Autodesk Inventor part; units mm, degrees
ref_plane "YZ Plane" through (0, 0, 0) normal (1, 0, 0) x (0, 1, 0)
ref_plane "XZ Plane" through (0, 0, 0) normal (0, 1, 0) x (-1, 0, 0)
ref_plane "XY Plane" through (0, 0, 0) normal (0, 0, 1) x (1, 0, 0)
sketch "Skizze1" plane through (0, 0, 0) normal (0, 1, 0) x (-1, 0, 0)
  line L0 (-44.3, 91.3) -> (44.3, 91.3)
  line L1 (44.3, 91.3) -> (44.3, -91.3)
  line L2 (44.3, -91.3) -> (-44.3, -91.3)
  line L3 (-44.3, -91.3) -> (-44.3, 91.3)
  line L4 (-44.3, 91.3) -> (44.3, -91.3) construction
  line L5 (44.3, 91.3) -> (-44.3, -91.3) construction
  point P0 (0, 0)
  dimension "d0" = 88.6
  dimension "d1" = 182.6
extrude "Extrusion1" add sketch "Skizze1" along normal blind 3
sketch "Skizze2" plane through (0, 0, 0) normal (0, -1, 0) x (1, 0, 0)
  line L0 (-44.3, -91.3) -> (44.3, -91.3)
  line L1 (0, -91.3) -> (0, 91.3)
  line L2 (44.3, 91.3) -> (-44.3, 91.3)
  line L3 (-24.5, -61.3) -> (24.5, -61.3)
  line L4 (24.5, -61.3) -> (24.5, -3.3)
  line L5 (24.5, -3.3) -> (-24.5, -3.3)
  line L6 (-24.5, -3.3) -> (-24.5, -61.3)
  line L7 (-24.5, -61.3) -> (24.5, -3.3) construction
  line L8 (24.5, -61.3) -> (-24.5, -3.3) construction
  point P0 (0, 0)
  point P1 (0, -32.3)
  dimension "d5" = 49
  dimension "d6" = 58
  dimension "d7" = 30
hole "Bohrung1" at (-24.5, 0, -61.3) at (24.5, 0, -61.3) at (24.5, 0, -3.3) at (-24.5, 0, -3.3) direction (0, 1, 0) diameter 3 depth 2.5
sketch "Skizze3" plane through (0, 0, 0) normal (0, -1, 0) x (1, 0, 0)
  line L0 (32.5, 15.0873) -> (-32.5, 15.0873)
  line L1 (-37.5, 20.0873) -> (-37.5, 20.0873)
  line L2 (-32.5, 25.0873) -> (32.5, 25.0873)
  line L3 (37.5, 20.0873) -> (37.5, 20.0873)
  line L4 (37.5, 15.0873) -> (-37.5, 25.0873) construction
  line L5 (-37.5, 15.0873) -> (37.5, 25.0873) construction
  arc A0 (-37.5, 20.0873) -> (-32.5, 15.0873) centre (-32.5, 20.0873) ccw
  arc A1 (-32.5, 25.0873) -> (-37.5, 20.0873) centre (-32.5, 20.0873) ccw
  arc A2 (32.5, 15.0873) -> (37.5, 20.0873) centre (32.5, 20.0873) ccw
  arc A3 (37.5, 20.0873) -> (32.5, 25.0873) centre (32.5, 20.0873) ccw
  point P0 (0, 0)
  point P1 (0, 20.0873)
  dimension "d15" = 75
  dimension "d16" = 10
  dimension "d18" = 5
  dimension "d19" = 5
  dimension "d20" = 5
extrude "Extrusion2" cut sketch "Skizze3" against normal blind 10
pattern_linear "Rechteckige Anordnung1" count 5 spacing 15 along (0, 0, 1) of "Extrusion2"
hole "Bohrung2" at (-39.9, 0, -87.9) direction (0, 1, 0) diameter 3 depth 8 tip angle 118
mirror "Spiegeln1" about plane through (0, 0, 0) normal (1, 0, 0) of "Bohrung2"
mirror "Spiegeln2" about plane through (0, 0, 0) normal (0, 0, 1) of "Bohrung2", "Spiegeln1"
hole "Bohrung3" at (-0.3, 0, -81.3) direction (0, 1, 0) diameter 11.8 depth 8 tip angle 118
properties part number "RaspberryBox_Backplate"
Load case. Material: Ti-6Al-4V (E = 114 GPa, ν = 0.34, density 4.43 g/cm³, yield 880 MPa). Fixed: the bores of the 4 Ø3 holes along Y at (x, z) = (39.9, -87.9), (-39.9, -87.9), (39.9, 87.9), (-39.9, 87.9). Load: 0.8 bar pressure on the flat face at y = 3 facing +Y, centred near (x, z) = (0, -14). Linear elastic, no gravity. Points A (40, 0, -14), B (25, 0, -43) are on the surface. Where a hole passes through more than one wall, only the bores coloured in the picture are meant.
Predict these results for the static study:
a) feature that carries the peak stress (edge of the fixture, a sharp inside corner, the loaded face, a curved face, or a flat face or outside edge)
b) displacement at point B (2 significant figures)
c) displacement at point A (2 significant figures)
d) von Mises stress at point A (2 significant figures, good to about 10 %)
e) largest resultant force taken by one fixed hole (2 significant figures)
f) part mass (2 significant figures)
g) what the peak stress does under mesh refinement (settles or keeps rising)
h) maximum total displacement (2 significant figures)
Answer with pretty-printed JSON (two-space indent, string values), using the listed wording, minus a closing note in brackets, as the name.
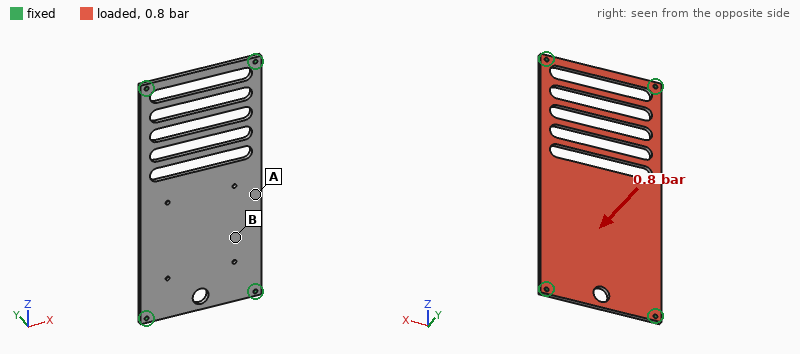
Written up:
{
  "feature that carries the peak stress": "edge of the fixture",
  "displacement at point B": "0.99 mm",
  "displacement at point A": "1.6 mm",
  "von Mises stress at point A": "70 MPa",
  "largest resultant force taken by one fixed hole": "310 N",
  "part mass": "160 g",
  "what the peak stress does under mesh refinement": "keeps rising",
  "maximum total displacement": "2.1 mm"
}
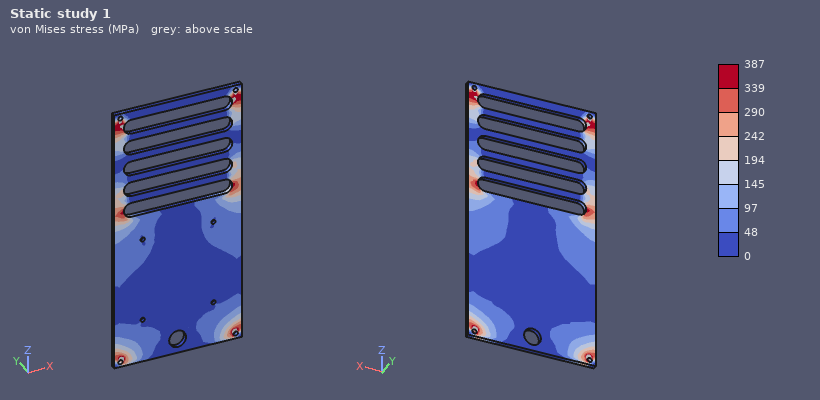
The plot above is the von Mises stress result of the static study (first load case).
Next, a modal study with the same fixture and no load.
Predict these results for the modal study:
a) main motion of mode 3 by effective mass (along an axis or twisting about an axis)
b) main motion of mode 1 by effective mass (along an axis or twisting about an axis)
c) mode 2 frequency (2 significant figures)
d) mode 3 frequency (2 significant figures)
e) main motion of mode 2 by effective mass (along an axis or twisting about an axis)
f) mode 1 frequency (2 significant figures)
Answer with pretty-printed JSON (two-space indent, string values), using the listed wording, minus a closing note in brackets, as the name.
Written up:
{
  "main motion of mode 3 by effective mass": "twisting about X",
  "main motion of mode 1 by effective mass": "along Y",
  "mode 2 frequency": "710 Hz",
  "mode 3 frequency": "990 Hz",
  "main motion of mode 2 by effective mass": "twisting about Z",
  "mode 1 frequency": "320 Hz"
}
